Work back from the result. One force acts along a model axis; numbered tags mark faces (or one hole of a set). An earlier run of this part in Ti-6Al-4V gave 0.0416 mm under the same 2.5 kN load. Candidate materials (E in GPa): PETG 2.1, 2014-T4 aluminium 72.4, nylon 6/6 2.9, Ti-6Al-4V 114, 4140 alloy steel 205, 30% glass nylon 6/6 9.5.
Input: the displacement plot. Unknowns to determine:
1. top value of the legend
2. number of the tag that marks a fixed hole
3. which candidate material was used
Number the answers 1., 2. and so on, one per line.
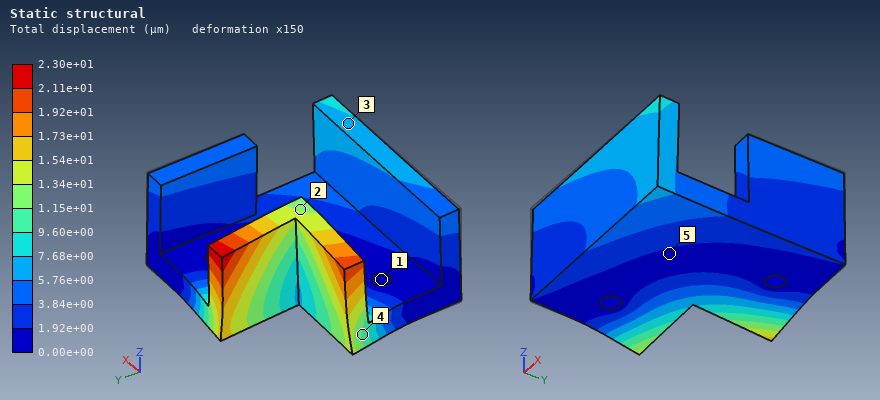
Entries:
1. 2.30e+01 µm
2. 1
3. 4140 alloy steel
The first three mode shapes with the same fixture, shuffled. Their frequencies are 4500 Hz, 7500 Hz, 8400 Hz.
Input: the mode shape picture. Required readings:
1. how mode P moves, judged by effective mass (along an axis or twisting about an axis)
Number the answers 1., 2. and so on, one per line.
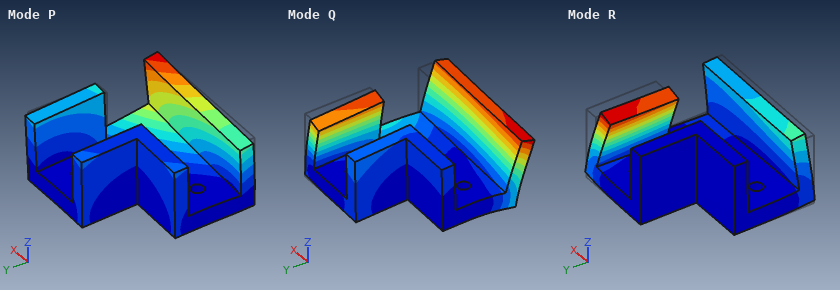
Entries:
1. along Z
